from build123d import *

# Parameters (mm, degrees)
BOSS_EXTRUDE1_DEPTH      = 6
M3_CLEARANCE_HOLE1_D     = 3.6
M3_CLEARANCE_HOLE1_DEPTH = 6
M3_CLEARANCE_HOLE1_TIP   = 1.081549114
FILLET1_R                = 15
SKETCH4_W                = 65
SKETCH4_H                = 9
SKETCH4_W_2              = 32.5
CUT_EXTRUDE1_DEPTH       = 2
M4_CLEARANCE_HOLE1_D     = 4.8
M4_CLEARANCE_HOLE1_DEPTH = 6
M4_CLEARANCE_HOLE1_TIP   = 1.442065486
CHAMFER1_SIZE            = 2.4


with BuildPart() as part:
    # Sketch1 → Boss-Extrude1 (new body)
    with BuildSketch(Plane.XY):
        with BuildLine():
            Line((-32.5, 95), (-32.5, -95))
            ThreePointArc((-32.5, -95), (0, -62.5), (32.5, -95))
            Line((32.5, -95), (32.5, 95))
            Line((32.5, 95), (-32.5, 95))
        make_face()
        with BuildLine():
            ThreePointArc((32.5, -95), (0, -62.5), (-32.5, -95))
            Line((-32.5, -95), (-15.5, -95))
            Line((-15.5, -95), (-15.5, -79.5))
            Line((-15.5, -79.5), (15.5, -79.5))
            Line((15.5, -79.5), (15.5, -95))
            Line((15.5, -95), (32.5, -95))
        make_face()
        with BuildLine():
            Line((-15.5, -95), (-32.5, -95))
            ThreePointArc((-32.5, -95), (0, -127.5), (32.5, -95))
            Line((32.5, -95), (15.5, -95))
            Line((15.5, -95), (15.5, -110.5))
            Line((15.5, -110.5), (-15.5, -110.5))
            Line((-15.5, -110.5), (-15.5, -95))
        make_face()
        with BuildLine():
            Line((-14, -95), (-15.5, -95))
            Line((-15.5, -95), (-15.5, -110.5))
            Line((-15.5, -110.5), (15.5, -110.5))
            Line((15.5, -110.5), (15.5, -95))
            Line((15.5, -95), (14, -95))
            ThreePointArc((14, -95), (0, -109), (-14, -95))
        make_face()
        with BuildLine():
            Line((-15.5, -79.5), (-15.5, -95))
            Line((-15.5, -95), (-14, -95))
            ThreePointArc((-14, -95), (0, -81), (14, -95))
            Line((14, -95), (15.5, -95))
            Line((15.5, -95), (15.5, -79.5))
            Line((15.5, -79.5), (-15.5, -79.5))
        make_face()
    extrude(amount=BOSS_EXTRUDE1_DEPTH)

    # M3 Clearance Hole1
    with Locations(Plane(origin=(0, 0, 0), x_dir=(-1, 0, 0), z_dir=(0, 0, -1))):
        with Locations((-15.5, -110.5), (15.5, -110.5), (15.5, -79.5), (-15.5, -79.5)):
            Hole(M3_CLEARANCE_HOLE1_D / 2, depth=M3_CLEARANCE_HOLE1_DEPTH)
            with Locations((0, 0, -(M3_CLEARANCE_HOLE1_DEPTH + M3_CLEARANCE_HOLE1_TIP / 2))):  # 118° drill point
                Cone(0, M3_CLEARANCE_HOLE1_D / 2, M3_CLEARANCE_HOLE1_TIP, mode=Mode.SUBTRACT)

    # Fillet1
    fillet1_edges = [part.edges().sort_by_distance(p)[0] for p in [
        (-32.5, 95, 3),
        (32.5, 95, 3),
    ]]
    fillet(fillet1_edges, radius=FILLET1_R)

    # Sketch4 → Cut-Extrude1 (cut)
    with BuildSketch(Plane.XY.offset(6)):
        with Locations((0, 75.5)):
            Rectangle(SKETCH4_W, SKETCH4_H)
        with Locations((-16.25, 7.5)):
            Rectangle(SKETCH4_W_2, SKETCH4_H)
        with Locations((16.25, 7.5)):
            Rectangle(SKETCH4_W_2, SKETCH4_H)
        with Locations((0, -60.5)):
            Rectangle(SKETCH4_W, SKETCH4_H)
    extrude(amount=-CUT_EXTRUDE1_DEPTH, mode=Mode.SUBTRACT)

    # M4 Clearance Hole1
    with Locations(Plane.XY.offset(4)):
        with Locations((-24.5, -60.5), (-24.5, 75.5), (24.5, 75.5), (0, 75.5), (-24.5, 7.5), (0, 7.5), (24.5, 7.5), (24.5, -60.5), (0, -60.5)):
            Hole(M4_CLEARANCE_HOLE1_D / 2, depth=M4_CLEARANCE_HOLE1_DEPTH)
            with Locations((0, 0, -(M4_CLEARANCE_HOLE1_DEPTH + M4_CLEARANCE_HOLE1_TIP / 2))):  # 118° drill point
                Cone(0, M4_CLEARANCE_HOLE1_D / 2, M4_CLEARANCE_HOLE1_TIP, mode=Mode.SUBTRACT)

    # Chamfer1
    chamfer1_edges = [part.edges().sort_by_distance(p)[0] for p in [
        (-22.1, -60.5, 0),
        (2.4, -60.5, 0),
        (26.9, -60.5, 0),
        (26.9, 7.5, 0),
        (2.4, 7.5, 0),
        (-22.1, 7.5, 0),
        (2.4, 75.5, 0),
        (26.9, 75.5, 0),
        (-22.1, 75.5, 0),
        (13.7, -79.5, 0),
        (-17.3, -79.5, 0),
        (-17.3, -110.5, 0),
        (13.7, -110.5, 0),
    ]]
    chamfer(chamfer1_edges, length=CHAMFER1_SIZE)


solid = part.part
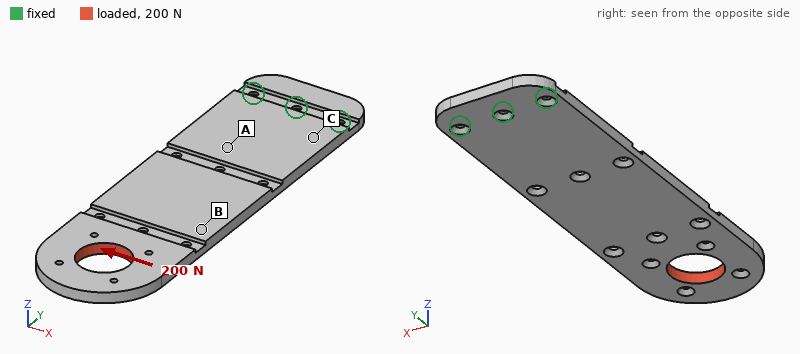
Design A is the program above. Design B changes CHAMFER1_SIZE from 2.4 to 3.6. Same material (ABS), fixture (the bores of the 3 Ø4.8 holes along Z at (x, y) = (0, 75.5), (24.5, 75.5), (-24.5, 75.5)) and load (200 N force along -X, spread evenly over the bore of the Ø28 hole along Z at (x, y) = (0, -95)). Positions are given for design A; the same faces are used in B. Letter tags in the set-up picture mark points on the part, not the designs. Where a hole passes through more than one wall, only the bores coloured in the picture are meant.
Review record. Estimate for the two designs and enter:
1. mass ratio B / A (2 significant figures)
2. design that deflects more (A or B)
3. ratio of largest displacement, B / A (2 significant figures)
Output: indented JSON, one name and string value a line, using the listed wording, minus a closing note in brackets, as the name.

{
  "mass ratio B / A": "0.99",
  "design that deflects more": "B",
  "ratio of largest displacement, B / A": "1.2"
}
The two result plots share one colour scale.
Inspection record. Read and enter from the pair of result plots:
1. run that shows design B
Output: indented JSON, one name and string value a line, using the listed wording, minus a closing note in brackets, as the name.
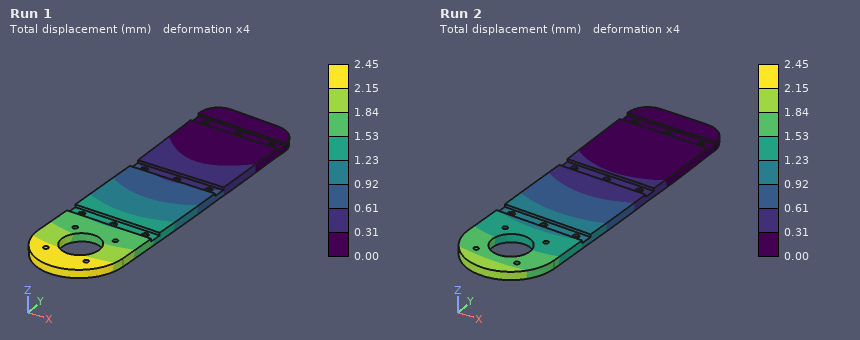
{
  "run that shows design B": "Run 1"
}
